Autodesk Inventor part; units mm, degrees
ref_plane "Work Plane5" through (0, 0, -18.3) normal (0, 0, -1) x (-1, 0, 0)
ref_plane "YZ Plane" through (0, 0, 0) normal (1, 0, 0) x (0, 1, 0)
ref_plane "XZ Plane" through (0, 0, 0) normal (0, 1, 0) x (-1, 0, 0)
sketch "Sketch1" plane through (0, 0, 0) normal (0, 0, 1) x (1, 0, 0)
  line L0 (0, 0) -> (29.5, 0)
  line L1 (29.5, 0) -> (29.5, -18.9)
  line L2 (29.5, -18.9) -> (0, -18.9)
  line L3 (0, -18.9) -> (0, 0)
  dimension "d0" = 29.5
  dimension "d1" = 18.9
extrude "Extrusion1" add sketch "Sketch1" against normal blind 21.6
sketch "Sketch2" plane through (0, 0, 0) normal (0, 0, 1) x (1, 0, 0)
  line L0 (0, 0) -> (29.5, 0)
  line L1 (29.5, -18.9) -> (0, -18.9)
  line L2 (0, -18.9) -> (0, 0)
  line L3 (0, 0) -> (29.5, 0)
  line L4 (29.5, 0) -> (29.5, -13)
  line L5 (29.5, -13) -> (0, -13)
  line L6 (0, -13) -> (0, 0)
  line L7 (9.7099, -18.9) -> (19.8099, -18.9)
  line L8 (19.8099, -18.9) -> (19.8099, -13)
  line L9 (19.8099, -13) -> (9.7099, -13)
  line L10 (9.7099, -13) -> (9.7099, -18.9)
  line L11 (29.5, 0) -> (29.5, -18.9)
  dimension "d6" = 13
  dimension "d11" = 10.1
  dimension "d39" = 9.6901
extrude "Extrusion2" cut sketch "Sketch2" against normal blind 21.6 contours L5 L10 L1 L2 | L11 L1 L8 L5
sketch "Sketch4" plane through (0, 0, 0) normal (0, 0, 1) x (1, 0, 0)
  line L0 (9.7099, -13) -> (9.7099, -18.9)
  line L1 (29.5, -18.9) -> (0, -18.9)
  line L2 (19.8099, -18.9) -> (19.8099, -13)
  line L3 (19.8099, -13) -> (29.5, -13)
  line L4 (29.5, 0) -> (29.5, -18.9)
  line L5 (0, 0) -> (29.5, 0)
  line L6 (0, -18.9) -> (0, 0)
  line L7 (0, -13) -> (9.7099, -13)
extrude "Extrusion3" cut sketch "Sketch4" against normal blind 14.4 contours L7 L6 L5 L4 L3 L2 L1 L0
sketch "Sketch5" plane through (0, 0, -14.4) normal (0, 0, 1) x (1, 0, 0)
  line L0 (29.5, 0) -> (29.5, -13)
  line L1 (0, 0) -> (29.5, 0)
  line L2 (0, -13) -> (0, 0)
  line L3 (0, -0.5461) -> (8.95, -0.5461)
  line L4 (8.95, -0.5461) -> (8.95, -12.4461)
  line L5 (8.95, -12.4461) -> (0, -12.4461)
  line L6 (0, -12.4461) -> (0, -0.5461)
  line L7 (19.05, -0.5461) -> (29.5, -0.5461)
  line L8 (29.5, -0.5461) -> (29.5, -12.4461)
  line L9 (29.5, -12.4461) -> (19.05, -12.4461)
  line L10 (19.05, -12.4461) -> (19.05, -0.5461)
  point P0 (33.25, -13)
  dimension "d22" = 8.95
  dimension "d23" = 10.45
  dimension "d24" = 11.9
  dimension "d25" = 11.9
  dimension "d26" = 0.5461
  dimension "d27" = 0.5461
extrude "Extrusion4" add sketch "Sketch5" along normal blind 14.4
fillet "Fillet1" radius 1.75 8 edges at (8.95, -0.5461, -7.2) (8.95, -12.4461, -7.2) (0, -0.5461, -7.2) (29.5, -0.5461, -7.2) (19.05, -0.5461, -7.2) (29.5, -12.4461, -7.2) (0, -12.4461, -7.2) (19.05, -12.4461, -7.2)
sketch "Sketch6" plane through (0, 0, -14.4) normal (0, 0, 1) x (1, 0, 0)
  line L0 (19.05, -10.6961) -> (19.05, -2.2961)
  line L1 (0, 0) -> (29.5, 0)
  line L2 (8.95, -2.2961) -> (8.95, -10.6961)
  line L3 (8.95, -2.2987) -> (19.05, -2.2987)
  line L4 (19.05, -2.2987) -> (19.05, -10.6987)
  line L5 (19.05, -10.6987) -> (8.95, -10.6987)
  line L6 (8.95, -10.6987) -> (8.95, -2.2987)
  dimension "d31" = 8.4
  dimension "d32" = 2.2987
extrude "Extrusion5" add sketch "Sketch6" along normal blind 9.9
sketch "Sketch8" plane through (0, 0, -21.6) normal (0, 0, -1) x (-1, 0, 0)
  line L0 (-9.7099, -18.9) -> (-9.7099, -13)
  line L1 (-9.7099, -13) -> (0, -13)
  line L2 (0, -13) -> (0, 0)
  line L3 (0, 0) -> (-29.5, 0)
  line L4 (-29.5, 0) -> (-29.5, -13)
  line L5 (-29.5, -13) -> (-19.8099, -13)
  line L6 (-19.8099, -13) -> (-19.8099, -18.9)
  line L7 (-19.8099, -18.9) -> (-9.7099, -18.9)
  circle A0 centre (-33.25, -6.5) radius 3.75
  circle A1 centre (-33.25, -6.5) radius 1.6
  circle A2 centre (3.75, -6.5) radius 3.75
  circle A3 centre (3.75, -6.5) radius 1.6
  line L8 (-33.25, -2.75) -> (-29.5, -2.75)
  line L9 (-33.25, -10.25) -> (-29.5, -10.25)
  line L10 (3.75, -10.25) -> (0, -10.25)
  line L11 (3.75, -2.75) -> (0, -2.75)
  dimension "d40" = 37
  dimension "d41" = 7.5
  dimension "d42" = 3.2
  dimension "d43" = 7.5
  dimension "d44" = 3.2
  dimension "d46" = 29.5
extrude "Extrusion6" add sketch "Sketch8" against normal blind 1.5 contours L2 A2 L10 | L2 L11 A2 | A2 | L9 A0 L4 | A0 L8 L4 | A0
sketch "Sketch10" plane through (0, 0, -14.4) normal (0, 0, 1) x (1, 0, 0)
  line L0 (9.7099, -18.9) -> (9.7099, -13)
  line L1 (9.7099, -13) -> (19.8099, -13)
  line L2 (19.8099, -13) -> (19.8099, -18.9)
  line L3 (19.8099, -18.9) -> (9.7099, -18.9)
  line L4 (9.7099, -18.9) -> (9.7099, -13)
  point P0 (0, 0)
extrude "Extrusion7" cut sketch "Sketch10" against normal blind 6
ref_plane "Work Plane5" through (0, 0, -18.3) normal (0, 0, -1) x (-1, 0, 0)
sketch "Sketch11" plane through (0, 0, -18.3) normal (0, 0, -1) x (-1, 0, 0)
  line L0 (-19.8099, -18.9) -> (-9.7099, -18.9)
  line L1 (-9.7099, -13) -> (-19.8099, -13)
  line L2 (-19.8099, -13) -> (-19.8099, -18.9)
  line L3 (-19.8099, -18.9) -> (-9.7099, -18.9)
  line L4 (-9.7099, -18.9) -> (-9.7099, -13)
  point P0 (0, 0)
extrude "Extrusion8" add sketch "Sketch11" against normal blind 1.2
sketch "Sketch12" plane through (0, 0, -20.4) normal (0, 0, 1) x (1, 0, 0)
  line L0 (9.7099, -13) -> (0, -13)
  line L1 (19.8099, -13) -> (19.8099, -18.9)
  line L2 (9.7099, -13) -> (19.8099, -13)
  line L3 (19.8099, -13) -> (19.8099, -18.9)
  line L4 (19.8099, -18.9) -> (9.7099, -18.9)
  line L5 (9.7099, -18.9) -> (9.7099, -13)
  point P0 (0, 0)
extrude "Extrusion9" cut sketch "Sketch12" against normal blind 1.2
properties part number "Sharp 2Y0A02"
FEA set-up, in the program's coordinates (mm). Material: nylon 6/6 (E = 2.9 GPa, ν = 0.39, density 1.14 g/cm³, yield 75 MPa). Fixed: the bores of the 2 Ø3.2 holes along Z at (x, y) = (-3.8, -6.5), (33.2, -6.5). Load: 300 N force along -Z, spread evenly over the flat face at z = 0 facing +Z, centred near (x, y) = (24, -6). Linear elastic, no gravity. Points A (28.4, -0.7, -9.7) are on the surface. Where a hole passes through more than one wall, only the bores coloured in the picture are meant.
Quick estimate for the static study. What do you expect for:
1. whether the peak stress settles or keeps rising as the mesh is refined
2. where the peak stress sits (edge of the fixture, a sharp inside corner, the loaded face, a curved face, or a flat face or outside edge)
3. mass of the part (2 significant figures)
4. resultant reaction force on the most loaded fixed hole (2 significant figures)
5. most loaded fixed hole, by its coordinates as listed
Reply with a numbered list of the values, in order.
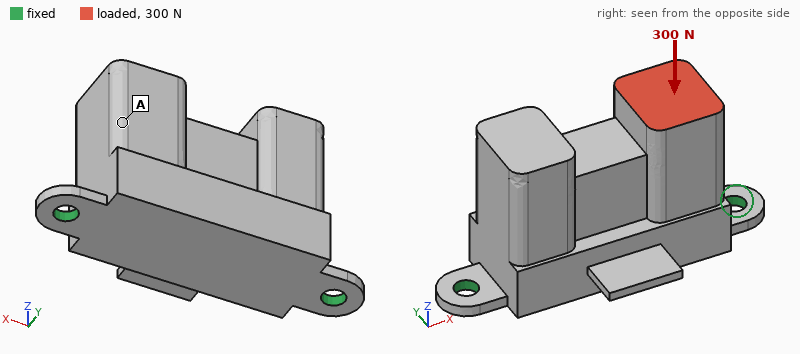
1. keeps rising
2. edge of the fixture
3. 8.0 g
4. 250 N
5. (33.2, -6.5)
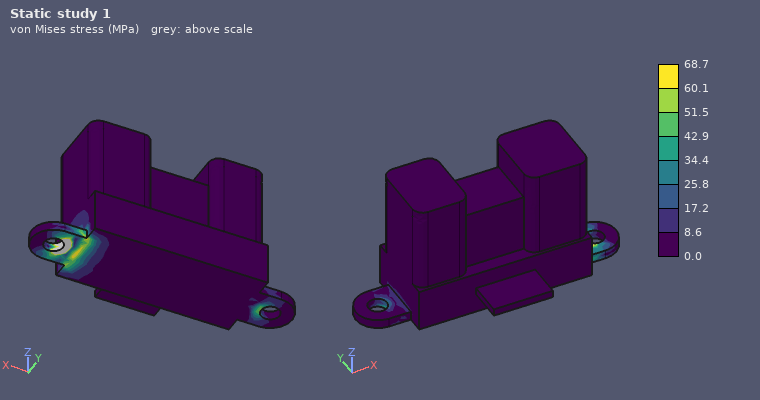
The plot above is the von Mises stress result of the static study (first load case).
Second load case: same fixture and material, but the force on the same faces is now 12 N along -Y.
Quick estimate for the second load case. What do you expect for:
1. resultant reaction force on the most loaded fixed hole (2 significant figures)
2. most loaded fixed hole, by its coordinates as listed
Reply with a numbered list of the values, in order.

1. 9.3 N
2. (33.2, -6.5)
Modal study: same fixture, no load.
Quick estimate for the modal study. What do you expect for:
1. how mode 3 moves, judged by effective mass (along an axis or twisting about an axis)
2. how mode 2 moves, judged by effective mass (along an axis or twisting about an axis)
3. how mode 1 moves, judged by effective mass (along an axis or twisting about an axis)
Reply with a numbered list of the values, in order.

1. along X
2. along Z
3. along Y
